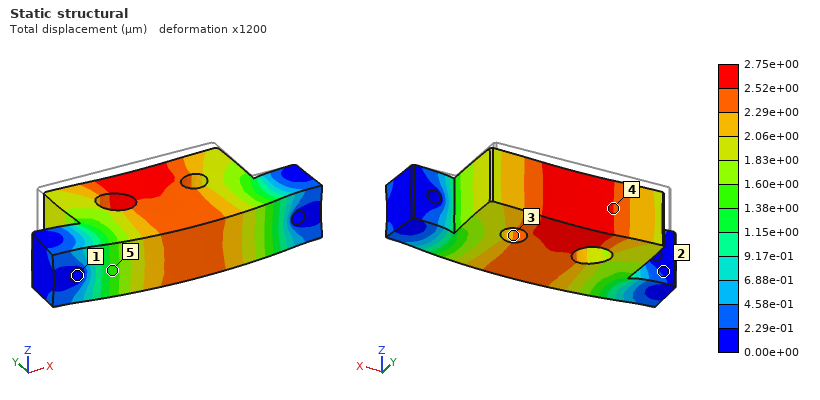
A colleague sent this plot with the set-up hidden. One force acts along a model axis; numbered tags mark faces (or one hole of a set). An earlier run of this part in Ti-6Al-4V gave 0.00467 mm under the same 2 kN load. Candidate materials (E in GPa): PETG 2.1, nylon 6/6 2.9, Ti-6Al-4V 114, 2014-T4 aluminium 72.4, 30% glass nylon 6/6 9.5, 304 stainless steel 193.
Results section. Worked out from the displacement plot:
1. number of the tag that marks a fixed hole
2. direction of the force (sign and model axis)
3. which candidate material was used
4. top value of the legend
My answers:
1
-Y
304 stainless steel
2.75e+00 µm
